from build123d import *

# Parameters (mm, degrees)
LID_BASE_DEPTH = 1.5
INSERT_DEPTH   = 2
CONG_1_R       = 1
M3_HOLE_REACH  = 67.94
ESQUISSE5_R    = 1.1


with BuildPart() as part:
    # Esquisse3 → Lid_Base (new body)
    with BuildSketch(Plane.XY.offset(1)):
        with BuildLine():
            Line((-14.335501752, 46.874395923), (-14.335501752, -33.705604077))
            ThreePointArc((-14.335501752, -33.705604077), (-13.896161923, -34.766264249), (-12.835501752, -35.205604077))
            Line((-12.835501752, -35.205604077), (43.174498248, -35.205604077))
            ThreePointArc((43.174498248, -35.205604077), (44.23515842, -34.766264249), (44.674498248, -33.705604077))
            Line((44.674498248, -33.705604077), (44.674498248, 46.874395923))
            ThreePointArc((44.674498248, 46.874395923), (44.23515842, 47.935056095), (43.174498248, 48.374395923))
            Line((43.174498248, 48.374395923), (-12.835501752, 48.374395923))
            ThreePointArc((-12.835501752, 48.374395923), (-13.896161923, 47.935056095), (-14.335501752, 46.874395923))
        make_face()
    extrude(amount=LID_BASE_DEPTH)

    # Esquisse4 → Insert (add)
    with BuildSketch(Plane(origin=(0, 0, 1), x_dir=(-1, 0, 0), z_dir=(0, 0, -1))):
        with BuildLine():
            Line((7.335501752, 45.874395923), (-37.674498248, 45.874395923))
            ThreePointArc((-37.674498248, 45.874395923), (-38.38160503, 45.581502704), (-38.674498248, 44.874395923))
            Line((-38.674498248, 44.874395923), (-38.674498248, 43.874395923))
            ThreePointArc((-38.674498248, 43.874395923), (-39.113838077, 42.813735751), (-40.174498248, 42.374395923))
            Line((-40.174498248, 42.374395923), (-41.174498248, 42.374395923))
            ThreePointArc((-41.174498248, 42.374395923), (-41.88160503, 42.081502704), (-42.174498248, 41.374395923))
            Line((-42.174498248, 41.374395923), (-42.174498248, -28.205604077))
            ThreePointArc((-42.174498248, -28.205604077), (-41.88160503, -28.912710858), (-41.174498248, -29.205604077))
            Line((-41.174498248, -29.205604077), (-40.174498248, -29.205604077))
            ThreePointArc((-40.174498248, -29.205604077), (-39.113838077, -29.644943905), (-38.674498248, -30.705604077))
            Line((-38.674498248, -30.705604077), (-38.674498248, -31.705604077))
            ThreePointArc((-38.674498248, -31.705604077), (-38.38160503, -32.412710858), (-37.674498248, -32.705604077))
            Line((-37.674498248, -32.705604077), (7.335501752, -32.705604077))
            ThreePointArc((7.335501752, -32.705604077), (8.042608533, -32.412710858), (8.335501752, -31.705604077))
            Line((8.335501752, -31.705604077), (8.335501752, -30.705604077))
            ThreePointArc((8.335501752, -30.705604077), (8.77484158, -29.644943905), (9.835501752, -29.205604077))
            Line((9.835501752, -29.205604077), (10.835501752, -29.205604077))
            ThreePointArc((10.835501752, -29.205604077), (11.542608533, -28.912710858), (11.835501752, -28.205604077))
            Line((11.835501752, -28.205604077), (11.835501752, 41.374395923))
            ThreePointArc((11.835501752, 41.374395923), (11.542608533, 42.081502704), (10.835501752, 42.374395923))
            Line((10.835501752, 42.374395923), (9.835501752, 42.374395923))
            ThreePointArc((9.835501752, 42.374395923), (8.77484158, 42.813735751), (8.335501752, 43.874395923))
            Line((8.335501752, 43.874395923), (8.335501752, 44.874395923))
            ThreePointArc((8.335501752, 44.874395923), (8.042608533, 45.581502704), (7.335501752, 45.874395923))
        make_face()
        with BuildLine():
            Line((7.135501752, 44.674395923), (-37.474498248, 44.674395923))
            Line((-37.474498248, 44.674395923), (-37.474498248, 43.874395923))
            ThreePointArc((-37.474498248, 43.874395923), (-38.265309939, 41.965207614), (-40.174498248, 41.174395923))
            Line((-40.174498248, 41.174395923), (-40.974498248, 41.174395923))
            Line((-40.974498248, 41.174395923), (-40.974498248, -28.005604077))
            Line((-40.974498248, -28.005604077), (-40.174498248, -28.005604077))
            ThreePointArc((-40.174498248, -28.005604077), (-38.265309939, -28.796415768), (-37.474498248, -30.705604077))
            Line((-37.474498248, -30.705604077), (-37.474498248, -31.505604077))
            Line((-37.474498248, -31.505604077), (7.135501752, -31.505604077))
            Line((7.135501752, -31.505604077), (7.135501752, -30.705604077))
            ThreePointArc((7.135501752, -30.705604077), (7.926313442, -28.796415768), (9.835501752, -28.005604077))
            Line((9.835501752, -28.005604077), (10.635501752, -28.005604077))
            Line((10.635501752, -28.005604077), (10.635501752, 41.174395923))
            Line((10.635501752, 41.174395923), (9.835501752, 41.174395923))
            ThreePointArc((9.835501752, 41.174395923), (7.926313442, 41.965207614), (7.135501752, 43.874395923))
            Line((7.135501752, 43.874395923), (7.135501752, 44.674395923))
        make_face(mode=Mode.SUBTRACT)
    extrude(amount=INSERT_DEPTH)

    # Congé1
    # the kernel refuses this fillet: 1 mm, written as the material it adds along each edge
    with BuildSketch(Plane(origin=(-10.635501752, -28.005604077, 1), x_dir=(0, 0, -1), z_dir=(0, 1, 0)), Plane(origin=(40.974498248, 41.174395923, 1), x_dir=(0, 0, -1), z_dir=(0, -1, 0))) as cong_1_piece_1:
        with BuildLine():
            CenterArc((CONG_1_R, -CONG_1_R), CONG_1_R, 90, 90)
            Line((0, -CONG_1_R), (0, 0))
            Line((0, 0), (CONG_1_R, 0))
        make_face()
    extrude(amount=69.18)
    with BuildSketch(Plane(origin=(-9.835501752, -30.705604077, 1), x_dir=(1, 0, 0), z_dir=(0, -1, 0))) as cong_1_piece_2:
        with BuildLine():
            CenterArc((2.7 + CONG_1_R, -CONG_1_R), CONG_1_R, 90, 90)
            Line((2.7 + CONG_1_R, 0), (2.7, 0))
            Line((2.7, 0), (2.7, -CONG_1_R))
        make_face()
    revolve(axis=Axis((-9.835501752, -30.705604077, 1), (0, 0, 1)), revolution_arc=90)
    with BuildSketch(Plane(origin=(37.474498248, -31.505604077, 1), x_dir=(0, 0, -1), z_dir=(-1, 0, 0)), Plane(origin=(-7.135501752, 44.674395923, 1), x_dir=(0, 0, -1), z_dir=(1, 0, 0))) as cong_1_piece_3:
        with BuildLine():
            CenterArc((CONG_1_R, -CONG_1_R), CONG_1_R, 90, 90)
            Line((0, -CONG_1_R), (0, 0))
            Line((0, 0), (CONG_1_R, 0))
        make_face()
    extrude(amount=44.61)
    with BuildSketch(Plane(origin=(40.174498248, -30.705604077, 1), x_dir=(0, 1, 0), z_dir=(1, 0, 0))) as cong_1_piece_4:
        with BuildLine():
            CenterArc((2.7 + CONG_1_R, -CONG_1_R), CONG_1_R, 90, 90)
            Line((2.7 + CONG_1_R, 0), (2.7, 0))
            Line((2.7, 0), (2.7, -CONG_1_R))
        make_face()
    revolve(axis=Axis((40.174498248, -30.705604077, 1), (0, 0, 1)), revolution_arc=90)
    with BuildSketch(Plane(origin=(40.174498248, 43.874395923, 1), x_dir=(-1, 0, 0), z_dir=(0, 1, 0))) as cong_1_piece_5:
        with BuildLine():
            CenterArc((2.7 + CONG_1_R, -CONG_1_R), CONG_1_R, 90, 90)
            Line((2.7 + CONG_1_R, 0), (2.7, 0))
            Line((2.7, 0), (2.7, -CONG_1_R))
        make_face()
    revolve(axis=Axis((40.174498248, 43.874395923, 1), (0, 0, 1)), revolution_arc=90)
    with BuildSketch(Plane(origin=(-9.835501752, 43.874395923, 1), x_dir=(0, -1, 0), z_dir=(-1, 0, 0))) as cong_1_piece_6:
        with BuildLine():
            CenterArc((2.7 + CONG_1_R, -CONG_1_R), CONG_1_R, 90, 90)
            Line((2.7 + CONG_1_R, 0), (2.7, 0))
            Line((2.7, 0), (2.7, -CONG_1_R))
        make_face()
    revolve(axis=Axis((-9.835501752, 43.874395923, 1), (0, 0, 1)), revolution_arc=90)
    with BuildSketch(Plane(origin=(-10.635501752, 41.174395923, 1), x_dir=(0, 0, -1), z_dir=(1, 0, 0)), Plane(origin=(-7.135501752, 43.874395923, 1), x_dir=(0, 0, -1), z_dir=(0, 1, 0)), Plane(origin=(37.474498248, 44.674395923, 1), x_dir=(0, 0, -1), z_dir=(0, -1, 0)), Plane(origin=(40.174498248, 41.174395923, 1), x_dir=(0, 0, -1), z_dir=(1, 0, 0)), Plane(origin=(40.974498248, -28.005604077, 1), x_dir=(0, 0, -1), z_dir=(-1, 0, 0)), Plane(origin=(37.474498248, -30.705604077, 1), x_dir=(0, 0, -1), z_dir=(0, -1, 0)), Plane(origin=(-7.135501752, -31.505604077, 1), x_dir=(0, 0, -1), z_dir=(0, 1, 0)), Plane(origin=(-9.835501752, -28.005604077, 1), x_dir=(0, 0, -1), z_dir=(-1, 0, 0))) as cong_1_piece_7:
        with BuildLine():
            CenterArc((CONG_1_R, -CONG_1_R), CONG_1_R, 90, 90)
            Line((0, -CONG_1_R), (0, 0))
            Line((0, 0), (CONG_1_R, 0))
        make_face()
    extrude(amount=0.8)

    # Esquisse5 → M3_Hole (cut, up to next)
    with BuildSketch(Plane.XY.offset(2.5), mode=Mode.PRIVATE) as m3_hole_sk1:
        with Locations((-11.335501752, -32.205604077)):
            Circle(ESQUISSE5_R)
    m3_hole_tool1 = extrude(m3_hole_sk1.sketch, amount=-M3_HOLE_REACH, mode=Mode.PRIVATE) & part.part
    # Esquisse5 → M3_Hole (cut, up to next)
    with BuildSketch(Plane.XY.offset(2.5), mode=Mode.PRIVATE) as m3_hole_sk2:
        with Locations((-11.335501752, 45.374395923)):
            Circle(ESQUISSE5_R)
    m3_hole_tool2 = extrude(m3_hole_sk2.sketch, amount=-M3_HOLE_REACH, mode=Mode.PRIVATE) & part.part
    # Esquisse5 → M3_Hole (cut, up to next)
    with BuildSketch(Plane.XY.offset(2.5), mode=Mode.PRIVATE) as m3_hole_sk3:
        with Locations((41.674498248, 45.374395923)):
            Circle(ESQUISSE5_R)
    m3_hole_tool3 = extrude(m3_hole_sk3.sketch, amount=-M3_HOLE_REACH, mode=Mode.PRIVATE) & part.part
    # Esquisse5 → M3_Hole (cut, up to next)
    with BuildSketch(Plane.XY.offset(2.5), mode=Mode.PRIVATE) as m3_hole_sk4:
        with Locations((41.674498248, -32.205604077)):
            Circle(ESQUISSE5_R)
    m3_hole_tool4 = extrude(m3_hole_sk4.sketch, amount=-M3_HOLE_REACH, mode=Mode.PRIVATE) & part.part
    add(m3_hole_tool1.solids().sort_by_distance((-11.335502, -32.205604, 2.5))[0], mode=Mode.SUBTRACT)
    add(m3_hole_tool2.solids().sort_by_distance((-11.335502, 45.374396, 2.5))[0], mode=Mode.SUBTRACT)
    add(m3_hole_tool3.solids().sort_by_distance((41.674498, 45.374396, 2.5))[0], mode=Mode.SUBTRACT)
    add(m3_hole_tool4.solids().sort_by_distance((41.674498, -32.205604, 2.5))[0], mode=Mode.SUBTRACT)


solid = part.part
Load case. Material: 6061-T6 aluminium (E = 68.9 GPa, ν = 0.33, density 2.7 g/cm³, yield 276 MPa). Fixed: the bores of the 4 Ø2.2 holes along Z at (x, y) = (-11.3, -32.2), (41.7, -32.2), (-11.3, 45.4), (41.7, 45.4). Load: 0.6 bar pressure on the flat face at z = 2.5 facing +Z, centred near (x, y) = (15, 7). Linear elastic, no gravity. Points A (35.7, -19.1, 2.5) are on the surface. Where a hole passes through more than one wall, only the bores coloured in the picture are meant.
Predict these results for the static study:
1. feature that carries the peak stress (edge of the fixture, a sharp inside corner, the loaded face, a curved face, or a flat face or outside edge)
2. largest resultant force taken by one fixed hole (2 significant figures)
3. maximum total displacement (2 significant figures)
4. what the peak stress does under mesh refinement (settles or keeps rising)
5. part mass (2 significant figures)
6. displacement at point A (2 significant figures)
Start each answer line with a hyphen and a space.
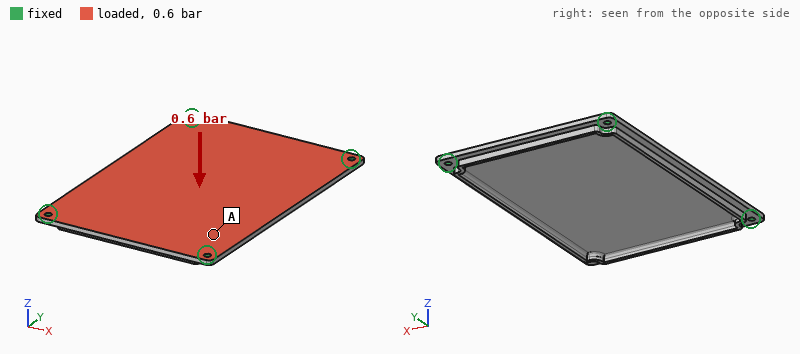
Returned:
- edge of the fixture
- 82 N
- 0.36 mm
- keeps rising
- 22 g
- 0.14 mm
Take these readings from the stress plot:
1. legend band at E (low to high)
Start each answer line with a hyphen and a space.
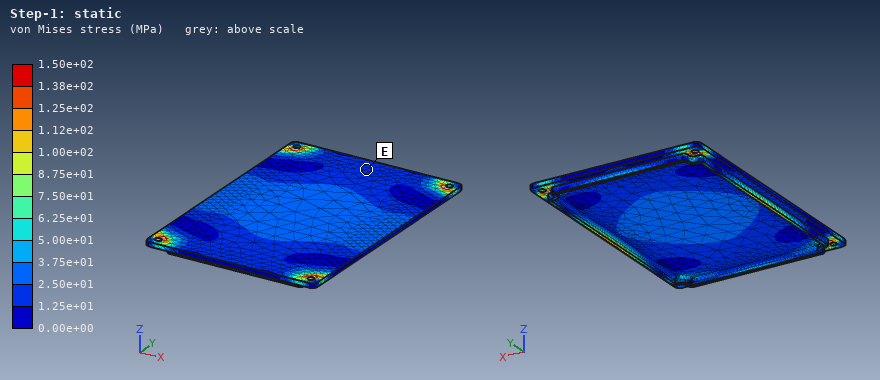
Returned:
- 1.25e+01 to 2.50e+01 MPa
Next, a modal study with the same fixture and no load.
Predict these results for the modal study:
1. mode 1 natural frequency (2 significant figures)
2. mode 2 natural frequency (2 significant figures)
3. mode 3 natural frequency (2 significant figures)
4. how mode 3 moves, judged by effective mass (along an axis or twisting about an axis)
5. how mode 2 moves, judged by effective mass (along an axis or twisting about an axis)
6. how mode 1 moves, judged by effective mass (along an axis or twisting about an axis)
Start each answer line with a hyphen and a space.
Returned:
- 1200 Hz
- 2000 Hz
- 2800 Hz
- twisting about X
- twisting about Y
- along Z
